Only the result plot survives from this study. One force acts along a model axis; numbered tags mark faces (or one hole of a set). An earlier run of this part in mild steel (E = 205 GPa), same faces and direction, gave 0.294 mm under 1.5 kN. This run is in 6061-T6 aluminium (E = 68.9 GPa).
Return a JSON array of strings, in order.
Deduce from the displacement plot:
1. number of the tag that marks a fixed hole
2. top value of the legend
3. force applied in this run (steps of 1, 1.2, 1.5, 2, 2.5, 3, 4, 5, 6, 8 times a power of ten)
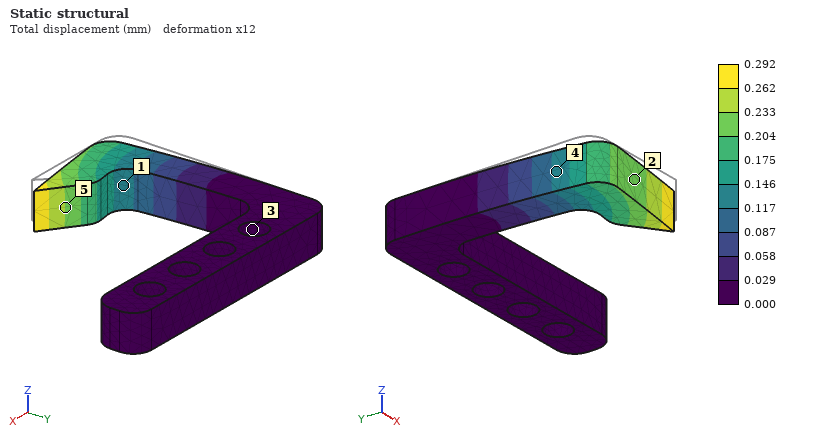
["3", "0.292 mm", "500 N"]
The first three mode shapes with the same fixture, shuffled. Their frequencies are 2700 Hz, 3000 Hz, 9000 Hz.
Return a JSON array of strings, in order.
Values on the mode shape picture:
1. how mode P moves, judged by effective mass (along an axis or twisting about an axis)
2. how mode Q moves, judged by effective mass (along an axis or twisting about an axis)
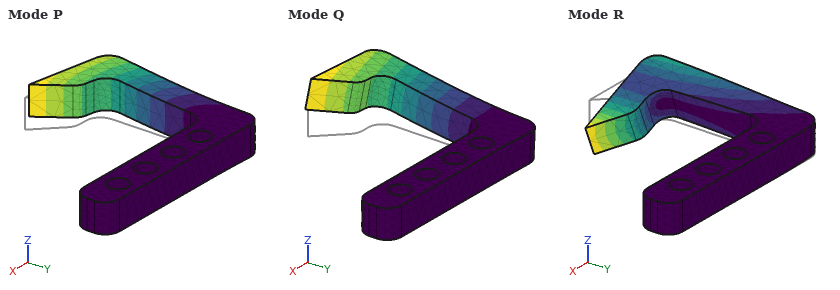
["along X", "along Z"]
